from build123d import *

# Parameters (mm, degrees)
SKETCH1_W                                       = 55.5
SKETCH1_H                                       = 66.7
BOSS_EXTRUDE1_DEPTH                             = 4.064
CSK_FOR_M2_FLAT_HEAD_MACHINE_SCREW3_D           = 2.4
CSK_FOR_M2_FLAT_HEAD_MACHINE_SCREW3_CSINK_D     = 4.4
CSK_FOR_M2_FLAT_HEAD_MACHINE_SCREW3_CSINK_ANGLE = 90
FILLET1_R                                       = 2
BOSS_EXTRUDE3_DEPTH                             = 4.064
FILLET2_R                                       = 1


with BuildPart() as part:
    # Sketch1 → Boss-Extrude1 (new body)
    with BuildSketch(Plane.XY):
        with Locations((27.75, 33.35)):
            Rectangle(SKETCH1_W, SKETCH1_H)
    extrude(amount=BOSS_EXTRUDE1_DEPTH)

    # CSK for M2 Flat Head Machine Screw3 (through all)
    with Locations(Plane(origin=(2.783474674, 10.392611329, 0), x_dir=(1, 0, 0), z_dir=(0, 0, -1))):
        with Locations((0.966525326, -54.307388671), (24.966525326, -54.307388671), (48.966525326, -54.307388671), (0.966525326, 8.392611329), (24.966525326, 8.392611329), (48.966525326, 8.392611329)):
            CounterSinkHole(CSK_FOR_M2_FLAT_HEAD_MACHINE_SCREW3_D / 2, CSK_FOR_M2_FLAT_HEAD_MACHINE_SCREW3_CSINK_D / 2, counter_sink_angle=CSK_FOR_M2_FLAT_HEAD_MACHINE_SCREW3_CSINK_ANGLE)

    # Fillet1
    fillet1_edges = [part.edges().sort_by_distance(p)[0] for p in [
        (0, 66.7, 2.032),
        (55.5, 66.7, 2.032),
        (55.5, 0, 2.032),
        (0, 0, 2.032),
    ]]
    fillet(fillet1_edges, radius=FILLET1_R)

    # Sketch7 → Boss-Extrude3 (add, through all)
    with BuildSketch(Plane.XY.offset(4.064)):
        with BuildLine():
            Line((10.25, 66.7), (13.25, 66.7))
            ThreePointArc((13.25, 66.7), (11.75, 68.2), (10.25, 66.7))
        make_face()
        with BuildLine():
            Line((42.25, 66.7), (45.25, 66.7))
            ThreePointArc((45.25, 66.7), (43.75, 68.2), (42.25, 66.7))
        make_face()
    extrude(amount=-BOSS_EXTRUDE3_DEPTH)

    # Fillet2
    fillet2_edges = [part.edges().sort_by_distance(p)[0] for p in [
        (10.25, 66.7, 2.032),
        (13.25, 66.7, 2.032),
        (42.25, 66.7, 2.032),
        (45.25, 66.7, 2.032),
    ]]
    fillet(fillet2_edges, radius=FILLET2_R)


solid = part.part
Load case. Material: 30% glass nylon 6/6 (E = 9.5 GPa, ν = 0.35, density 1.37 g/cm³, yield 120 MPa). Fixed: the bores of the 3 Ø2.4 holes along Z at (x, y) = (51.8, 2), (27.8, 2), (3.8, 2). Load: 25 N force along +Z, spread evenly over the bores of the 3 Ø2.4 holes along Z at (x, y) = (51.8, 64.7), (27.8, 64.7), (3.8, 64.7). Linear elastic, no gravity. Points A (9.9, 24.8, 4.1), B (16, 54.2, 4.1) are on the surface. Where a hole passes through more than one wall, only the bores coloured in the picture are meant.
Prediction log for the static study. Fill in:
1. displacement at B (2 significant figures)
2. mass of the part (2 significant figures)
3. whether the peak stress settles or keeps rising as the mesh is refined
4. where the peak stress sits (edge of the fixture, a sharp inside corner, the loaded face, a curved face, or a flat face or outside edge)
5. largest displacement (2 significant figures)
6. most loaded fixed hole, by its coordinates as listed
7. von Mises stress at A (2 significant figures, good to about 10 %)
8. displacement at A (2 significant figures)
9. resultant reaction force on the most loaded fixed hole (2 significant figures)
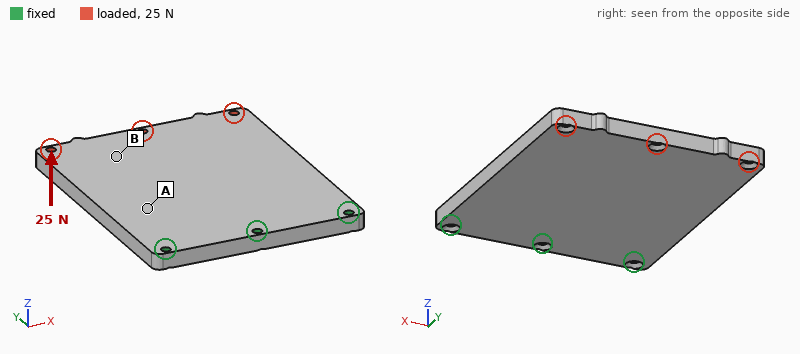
0.70 mm
20 g
keeps rising
edge of the fixture
0.97 mm
(27.8, 2)
6.4 MPa
0.20 mm
24 N
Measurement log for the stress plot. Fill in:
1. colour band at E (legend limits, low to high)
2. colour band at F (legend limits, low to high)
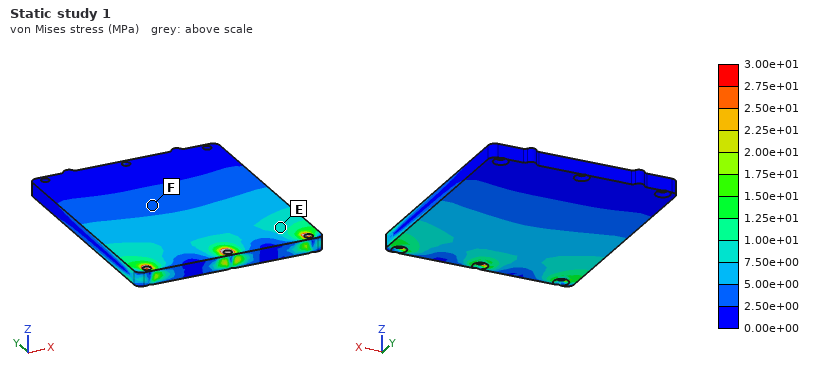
7.50e+00 to 1.00e+01 MPa
2.50e+00 to 5.00e+00 MPa
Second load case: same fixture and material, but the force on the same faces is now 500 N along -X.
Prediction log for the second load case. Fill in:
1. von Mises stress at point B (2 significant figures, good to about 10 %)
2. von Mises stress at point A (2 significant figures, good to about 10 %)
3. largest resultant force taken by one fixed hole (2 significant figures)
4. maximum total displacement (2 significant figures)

6.4 MPa
8.1 MPa
670 N
0.20 mm
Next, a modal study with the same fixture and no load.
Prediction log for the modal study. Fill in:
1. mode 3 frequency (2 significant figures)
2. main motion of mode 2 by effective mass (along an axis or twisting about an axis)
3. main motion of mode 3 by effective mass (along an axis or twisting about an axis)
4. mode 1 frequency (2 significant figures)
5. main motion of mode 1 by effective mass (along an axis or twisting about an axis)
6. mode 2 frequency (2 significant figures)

2300 Hz
twisting about Y
along Z
350 Hz
along Z
1100 Hz
